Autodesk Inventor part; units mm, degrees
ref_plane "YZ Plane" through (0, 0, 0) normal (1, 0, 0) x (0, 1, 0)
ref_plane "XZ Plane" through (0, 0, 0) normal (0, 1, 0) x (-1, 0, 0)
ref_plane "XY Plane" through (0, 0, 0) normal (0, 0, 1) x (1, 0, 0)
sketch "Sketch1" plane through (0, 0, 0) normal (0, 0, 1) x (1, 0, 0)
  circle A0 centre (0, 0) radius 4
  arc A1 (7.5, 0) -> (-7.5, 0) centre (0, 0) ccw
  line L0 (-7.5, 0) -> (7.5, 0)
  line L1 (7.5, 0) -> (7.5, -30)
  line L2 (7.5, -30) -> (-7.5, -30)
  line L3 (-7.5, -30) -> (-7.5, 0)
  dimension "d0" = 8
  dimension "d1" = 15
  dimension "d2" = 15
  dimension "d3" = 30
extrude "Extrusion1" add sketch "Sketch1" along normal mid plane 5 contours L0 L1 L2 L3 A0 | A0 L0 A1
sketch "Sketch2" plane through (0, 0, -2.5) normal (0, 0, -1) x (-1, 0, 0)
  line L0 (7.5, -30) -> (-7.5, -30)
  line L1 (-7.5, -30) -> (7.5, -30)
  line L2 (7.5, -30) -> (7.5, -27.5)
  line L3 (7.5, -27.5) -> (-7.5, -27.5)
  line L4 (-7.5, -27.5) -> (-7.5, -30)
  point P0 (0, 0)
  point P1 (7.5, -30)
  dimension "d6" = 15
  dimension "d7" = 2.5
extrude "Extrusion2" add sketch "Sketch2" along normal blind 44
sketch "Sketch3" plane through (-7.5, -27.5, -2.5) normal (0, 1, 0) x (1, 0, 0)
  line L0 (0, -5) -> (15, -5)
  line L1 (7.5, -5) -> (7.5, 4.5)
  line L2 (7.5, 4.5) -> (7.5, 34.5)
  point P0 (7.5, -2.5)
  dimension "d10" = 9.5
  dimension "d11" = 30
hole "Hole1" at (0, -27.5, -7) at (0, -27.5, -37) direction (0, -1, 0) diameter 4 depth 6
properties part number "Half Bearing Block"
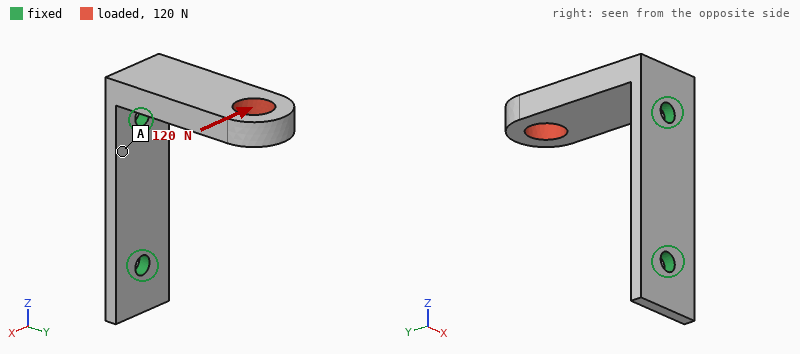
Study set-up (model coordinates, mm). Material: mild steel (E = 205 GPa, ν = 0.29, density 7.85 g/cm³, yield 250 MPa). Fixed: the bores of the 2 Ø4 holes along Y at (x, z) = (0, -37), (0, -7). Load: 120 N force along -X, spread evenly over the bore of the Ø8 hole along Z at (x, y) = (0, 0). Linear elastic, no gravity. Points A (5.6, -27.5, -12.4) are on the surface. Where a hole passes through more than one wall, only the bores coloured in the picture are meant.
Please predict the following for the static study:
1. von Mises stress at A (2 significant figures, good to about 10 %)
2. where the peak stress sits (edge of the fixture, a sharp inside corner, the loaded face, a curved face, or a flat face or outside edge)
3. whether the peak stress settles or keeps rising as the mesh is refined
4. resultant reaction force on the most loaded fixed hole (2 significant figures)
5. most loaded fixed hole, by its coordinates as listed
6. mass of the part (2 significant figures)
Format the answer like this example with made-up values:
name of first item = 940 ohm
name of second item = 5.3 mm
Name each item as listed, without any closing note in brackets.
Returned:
von Mises stress at A = 25 MPa
where the peak stress sits = edge of the fixture
whether the peak stress settles or keeps rising as the mesh is refined = keeps rising
resultant reaction force on the most loaded fixed hole = 130 N
most loaded fixed hole, by its coordinates as listed = (0, -7)
mass of the part = 32 g
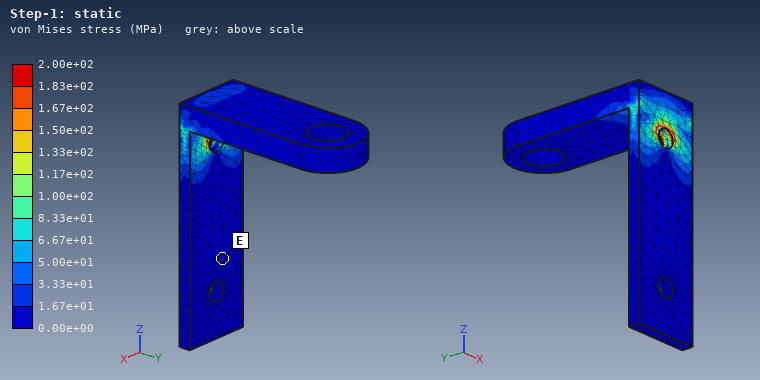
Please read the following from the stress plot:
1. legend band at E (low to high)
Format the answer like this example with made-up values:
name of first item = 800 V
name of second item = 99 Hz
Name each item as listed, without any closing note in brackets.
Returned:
legend band at E = 0.00e+00 to 1.67e+01 MPa
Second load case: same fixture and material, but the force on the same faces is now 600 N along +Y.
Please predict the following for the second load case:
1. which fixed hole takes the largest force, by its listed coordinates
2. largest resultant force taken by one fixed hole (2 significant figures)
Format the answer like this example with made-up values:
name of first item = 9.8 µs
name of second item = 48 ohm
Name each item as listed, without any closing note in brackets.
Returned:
which fixed hole takes the largest force, by its listed coordinates = (0, -7)
largest resultant force taken by one fixed hole = 610 N
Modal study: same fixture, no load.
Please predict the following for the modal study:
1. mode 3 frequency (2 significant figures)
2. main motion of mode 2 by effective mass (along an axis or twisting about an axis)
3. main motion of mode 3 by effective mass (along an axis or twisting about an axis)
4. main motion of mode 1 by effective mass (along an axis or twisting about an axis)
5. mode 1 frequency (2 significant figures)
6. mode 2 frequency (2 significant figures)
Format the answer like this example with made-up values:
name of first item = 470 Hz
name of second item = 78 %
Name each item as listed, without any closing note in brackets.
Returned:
mode 3 frequency = 11 kHz
main motion of mode 2 by effective mass = along X
main motion of mode 3 by effective mass = along Y
main motion of mode 1 by effective mass = along Z
mode 1 frequency = 1600 Hz
mode 2 frequency = 2600 Hz
